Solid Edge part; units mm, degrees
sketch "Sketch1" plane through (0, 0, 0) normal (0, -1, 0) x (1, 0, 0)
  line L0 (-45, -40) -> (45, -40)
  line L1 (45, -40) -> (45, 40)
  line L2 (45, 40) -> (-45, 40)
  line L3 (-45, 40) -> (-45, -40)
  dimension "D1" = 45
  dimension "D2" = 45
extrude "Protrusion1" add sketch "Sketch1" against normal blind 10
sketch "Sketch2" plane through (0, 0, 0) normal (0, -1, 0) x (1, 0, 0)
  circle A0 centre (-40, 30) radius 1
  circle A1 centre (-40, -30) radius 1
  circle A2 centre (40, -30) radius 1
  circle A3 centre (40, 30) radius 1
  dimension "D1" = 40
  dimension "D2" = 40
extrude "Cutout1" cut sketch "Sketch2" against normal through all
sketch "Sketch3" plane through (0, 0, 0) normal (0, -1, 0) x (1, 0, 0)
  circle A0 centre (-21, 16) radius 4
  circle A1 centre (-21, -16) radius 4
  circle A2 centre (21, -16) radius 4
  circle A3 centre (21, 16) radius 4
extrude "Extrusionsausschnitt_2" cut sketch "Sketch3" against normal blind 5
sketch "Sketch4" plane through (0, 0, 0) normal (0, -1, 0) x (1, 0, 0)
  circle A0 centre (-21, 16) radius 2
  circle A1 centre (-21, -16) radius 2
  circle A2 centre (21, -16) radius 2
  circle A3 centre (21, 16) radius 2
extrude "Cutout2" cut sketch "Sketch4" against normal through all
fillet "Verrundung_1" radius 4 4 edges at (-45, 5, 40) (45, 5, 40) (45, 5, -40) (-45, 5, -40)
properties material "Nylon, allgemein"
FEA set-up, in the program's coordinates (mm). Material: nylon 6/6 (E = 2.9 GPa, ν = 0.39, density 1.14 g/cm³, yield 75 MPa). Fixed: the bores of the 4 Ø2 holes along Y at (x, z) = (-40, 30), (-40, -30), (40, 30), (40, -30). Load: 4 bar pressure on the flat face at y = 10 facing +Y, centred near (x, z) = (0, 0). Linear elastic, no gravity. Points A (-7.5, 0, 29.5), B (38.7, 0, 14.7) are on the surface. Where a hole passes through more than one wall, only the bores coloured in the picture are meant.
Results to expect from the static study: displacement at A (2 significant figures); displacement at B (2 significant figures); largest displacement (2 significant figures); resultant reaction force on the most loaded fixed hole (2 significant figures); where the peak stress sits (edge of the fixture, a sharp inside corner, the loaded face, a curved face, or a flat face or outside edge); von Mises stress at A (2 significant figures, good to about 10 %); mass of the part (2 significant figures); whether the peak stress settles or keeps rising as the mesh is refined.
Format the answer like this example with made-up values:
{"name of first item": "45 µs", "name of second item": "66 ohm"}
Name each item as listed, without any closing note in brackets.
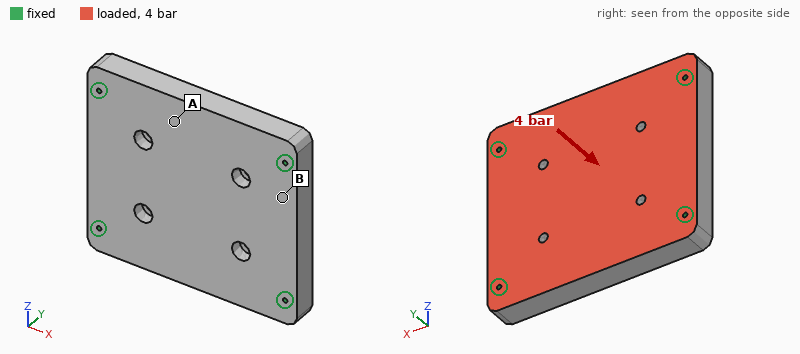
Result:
{"displacement at A": "0.40 mm", "displacement at B": "0.14 mm", "largest displacement": "0.47 mm", "resultant reaction force on the most loaded fixed hole": "710 N", "where the peak stress sits": "edge of the fixture", "von Mises stress at A": "9.2 MPa", "mass of the part": "80 g", "whether the peak stress settles or keeps rising as the mesh is refined": "keeps rising"}
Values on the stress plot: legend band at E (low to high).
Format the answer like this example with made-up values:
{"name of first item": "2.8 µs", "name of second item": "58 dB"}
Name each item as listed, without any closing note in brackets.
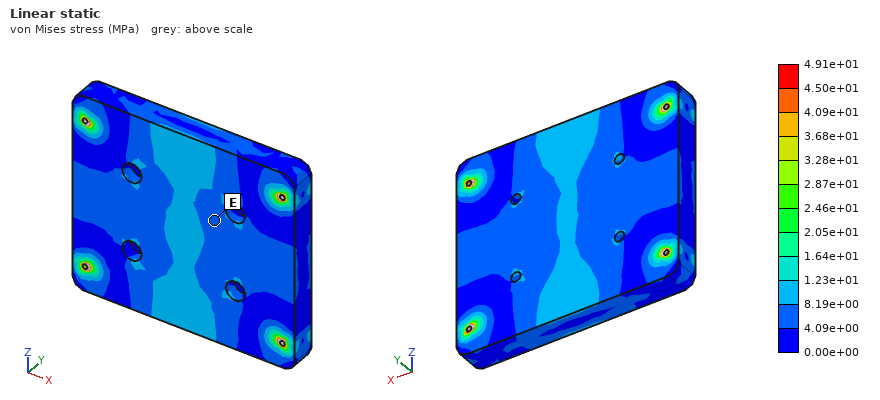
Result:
{"legend band at E": "4.09e+00 to 8.19e+00 MPa"}
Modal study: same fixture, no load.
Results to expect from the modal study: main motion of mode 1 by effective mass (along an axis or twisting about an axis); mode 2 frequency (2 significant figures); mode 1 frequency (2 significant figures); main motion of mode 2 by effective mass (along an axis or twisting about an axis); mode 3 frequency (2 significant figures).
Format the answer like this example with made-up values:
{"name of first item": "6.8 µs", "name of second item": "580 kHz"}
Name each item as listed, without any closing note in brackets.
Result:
{"main motion of mode 1 by effective mass": "along Y", "mode 2 frequency": "2300 Hz", "mode 1 frequency": "1600 Hz", "main motion of mode 2 by effective mass": "twisting about X", "mode 3 frequency": "3100 Hz"}
